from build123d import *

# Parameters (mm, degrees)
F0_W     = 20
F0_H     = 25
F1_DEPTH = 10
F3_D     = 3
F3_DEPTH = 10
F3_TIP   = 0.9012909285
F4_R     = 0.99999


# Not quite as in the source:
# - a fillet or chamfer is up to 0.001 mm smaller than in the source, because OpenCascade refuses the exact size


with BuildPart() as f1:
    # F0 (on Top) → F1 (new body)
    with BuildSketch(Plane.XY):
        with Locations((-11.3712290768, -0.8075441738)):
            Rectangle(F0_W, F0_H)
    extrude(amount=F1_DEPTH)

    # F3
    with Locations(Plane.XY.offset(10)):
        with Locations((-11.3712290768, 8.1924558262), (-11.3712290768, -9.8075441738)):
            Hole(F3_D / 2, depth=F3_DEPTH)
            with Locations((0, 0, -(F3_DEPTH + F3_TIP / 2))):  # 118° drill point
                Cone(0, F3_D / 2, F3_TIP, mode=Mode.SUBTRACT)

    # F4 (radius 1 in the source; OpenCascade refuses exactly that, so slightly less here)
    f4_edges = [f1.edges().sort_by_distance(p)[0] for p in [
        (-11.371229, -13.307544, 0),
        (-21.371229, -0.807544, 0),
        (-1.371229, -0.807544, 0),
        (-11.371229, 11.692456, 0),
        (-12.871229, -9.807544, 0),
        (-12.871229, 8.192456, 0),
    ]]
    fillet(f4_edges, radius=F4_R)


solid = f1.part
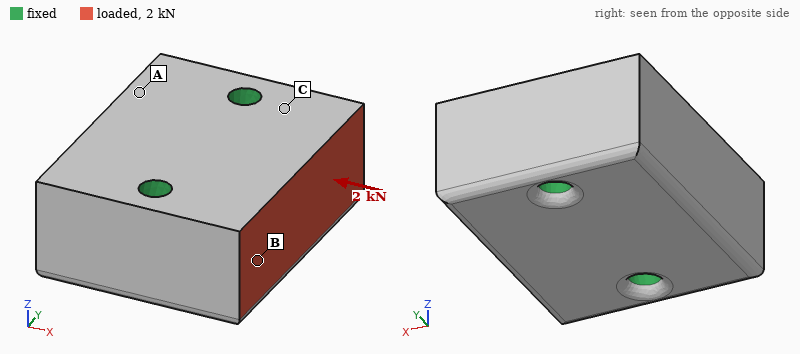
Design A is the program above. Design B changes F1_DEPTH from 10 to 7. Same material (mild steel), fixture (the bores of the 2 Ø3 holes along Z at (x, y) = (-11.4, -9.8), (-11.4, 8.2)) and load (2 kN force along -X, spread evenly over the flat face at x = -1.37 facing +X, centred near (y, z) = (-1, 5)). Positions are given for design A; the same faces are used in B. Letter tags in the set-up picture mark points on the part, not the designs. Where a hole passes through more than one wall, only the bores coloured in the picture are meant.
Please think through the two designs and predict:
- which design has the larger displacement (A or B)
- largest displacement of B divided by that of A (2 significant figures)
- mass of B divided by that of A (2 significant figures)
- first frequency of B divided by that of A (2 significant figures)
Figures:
B
1.6
0.70
0.81
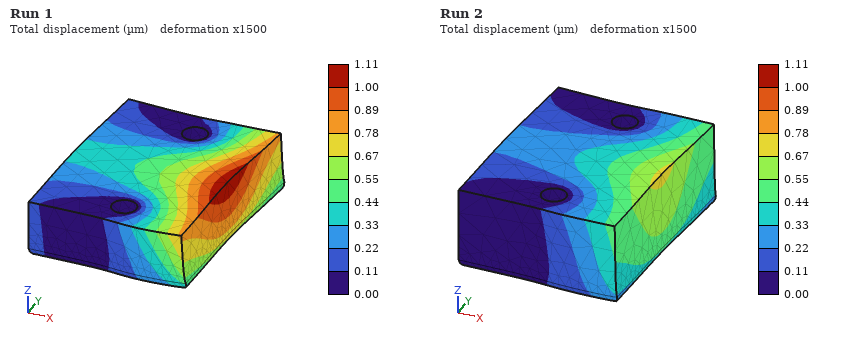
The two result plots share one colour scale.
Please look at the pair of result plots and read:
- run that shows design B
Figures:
Run 1
